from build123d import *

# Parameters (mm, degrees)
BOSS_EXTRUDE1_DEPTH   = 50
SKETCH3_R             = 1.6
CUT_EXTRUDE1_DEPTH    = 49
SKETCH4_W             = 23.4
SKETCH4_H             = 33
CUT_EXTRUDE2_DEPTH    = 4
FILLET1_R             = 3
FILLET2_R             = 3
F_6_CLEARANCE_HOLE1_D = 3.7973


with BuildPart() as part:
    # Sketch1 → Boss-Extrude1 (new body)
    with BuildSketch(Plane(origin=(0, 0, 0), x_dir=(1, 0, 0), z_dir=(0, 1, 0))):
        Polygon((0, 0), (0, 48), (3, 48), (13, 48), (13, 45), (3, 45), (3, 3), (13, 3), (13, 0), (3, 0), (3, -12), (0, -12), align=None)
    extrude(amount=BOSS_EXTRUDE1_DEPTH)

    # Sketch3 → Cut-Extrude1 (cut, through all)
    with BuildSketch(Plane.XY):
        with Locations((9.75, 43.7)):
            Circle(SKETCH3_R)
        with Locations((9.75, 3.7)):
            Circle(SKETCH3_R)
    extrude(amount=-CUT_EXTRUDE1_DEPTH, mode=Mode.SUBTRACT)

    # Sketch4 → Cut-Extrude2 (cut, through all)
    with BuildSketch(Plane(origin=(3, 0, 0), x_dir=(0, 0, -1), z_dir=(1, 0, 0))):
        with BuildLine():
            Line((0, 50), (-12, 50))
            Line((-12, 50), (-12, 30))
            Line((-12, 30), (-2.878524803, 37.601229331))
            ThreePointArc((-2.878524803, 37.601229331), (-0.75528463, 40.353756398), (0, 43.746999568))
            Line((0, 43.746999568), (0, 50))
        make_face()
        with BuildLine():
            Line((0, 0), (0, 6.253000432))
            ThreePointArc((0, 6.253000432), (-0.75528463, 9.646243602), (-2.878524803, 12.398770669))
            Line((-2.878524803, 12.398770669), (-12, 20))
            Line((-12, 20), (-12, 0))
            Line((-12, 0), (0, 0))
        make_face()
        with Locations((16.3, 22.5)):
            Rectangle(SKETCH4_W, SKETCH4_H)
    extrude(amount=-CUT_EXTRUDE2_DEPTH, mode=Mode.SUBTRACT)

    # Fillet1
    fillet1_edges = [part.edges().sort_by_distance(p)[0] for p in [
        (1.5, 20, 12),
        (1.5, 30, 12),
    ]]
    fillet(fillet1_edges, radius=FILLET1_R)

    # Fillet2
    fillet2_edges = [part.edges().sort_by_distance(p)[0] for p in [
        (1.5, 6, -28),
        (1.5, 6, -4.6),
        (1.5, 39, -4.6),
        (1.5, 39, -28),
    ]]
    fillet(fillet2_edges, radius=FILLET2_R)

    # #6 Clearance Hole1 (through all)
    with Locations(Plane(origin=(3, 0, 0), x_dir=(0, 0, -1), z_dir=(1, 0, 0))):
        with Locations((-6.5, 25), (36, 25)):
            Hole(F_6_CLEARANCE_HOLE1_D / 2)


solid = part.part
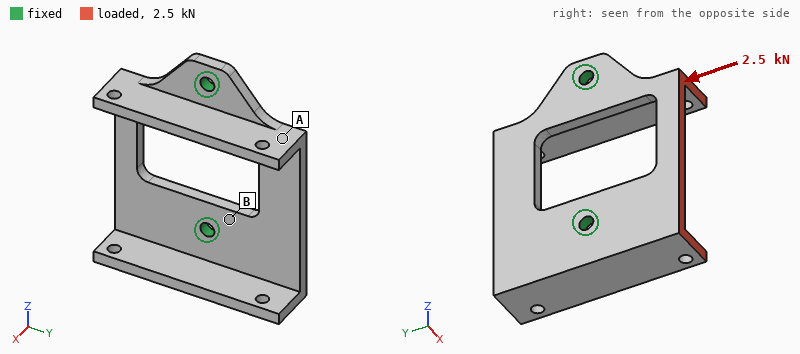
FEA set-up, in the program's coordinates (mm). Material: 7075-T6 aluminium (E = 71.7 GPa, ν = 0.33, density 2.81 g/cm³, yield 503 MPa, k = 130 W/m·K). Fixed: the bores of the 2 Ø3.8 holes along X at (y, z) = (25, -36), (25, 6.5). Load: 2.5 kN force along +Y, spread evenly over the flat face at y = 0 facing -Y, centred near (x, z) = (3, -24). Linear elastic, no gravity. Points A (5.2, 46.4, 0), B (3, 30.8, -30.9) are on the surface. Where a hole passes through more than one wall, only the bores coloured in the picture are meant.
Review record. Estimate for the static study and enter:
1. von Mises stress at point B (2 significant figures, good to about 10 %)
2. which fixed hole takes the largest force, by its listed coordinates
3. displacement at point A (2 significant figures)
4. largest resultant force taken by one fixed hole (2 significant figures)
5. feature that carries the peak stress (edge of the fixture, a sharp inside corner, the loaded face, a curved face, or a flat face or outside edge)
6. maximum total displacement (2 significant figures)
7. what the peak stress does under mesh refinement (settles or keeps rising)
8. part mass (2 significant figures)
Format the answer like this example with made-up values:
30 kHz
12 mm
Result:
31 MPa
(25, -36)
56 µm
1.7 kN
edge of the fixture
95 µm
keeps rising
24 g
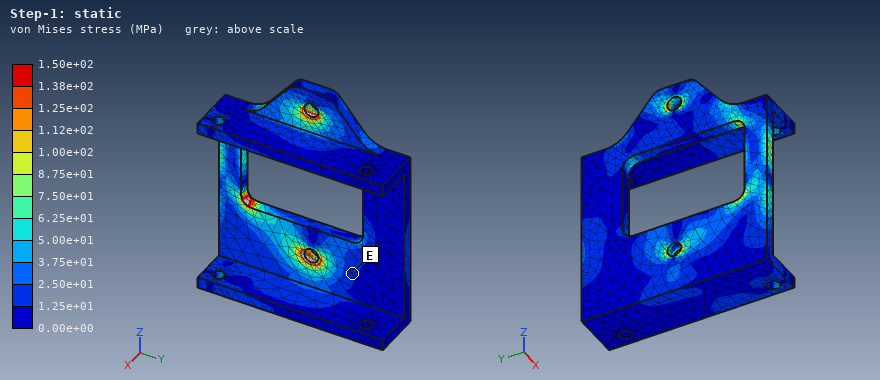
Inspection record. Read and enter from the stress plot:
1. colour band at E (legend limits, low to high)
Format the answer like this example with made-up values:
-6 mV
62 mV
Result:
1.25e+01 to 2.50e+01 MPa
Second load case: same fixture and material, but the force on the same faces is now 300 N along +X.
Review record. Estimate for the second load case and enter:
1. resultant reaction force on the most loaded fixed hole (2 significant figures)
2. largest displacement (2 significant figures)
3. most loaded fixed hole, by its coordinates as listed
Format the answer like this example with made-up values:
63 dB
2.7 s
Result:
180 N
0.17 mm
(25, -36)
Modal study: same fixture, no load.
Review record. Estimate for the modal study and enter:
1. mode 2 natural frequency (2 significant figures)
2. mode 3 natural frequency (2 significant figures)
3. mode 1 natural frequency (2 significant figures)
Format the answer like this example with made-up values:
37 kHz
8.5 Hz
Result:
3900 Hz
4800 Hz
2800 Hz
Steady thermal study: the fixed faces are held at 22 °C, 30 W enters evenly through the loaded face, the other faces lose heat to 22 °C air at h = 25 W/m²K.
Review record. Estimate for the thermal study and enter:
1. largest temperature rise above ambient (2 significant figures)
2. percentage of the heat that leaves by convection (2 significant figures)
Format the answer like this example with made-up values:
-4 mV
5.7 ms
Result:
61 K
9.4 %
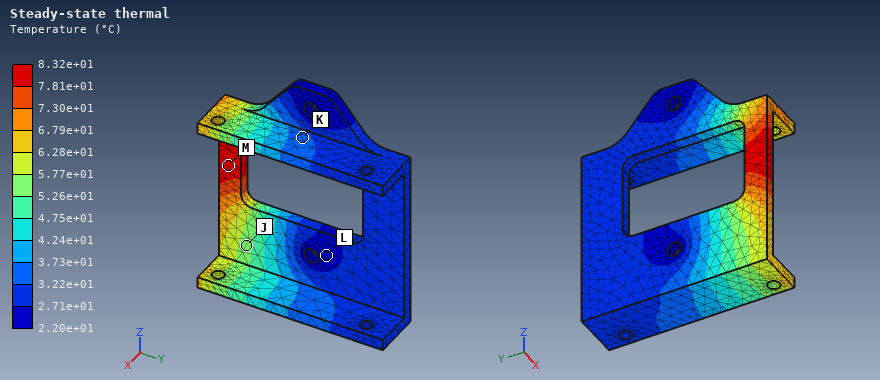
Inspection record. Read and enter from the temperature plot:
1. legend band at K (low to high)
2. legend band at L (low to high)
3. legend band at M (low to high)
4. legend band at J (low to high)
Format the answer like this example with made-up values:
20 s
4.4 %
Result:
3.22e+01 to 3.73e+01 °C
2.20e+01 to 2.71e+01 °C
7.81e+01 to 8.32e+01 °C
5.26e+01 to 5.77e+01 °C
